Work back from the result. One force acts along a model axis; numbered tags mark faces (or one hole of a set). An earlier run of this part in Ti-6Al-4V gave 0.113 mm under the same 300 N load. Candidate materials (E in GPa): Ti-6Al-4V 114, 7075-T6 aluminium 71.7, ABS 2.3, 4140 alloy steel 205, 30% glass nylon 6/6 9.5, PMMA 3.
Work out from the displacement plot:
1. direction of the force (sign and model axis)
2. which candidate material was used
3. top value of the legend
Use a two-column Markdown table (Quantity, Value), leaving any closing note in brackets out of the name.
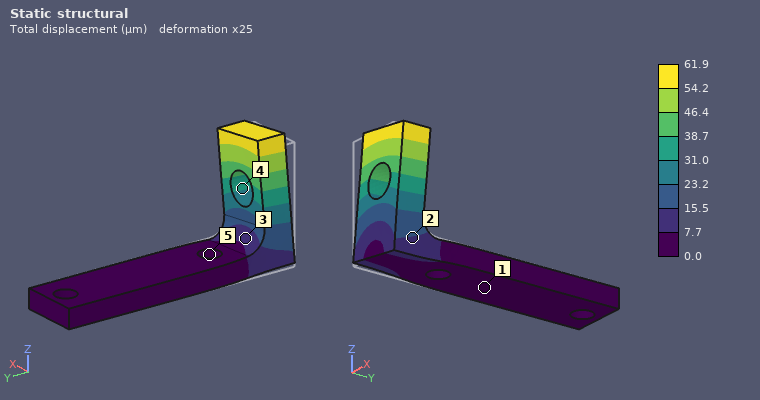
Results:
| Quantity | Value |
|---|---|
| direction of the force | +X |
| which candidate material was used | 4140 alloy steel |
| top value of the legend | 61.9 µm |
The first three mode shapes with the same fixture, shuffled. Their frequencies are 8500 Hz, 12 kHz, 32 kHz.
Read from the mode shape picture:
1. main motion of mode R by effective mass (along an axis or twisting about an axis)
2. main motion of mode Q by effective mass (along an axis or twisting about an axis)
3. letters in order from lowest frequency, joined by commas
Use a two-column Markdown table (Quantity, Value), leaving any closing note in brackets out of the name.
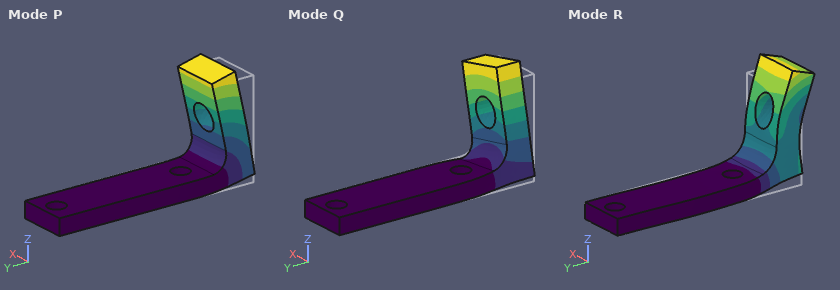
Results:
| Quantity | Value |
|---|---|
| main motion of mode R by effective mass | along Z |
| main motion of mode Q by effective mass | along X |
| letters in order from lowest frequency, joined by commas | P, Q, R |
